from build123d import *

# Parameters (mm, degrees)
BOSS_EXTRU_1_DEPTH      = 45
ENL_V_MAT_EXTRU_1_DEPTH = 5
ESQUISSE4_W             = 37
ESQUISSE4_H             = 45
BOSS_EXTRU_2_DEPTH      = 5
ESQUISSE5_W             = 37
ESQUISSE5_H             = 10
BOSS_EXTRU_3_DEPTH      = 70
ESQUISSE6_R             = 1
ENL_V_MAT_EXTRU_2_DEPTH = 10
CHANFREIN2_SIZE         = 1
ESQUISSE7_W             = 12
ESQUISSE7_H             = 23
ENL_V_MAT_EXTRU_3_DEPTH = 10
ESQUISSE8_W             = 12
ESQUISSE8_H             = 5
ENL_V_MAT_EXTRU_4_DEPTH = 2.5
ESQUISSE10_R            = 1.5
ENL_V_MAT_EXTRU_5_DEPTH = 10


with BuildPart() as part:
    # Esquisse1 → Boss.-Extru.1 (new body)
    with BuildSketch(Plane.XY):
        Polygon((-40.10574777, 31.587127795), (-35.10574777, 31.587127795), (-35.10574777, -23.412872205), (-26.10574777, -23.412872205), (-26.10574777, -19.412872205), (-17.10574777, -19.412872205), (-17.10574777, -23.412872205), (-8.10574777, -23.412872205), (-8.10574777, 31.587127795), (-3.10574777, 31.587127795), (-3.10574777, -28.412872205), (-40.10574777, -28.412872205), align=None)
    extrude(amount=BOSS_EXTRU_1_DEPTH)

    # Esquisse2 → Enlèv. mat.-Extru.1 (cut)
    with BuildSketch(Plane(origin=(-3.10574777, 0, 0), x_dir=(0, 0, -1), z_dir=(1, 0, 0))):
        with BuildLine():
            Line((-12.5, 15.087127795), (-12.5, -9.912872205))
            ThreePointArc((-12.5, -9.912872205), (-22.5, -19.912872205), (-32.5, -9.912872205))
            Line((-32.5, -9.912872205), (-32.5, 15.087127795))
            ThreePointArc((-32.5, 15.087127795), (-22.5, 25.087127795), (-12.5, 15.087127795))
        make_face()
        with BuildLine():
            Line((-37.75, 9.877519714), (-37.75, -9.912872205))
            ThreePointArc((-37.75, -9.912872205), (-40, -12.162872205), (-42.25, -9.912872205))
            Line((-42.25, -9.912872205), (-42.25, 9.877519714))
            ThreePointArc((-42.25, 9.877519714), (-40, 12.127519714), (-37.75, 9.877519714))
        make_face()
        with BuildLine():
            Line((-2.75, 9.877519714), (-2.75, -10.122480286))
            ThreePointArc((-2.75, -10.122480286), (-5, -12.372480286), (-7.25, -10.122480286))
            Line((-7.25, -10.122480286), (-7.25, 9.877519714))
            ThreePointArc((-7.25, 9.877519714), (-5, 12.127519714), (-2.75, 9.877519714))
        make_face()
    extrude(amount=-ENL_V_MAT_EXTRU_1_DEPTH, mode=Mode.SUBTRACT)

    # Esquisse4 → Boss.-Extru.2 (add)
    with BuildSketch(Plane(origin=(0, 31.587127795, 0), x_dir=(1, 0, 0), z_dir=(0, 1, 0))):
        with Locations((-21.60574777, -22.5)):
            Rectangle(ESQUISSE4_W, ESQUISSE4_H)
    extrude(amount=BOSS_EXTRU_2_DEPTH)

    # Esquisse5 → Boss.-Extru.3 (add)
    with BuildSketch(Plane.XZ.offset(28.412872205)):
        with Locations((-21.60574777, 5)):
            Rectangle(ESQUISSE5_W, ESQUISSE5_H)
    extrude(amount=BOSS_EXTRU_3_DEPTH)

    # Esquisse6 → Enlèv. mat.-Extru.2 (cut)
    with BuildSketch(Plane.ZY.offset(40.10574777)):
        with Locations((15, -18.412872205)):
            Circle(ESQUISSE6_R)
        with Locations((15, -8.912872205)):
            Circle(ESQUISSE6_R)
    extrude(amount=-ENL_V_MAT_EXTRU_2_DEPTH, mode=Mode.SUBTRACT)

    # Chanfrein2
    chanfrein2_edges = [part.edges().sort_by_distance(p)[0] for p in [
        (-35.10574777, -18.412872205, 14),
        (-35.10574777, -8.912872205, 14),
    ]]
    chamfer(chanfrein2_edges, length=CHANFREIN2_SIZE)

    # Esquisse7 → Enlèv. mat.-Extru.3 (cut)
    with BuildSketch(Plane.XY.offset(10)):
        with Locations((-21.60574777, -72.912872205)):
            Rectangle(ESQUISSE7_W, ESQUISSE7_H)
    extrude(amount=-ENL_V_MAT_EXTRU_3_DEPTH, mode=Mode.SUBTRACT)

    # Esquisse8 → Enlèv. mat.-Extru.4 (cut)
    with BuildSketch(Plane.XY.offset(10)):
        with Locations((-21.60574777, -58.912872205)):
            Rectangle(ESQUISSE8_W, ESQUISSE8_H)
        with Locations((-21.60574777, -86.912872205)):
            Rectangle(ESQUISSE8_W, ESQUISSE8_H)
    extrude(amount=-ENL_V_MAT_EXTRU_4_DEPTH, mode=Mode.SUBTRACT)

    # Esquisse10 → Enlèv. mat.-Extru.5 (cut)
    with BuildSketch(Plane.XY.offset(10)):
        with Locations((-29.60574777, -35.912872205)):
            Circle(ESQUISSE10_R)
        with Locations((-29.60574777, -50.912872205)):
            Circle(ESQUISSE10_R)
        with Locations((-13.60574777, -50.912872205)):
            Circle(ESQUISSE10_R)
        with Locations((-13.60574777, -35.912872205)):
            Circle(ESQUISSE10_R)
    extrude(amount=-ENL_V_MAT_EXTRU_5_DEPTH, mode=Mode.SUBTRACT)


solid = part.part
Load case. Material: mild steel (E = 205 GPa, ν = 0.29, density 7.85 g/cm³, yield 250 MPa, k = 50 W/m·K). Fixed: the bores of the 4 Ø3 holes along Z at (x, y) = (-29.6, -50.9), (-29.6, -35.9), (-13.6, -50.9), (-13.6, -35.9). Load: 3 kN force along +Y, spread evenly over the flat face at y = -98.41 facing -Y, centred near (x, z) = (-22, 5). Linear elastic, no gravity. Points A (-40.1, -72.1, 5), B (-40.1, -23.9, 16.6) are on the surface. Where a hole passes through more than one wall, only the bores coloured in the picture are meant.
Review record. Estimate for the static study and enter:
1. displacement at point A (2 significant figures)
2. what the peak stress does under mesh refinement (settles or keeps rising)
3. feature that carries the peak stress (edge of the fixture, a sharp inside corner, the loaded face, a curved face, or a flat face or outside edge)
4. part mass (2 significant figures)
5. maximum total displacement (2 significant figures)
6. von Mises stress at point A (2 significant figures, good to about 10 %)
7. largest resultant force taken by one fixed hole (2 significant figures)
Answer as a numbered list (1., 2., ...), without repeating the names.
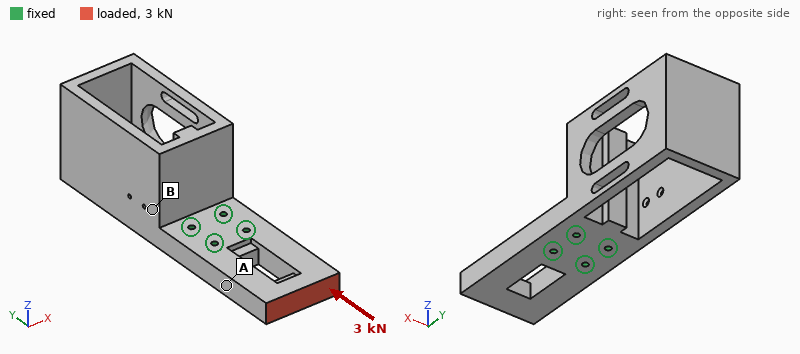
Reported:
1. 1.7 µm
2. keeps rising
3. edge of the fixture
4. 470 g
5. 3.5 µm
6. 7.2 MPa
7. 1.1 kN
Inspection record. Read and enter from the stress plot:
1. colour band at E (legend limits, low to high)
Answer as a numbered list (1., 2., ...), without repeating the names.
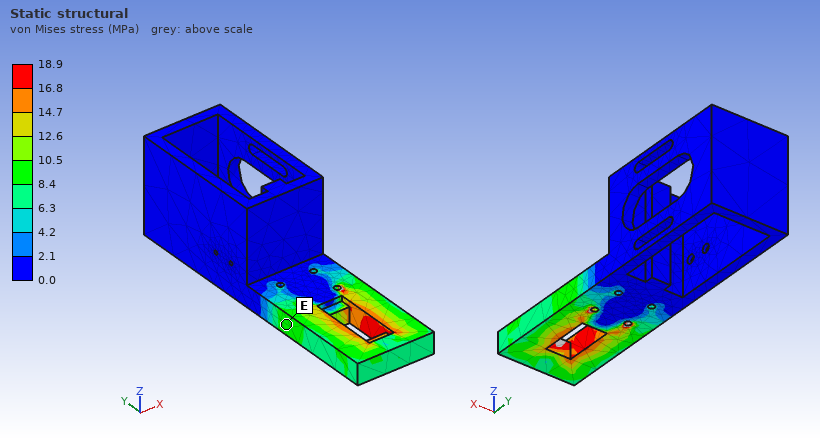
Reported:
1. 8.4 to 10.5 MPa
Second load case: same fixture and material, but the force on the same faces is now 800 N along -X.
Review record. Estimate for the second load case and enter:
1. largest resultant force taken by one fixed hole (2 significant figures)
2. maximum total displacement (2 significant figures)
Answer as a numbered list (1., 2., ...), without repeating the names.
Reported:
1. 1.2 kN
2. 13 µm
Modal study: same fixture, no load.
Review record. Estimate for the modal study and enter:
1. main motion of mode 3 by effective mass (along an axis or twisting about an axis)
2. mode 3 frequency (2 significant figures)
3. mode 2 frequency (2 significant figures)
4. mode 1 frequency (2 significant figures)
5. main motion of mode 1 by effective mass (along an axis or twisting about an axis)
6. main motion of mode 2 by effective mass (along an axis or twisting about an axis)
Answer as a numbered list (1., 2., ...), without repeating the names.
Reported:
1. twisting about Y
2. 2200 Hz
3. 1100 Hz
4. 1000 Hz
5. along Z
6. along X
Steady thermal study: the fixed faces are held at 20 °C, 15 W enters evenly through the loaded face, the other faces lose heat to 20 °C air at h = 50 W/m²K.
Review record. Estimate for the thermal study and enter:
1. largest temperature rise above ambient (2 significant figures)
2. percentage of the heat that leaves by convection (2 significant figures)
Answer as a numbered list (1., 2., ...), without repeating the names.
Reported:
1. 42 K
2. 32 %
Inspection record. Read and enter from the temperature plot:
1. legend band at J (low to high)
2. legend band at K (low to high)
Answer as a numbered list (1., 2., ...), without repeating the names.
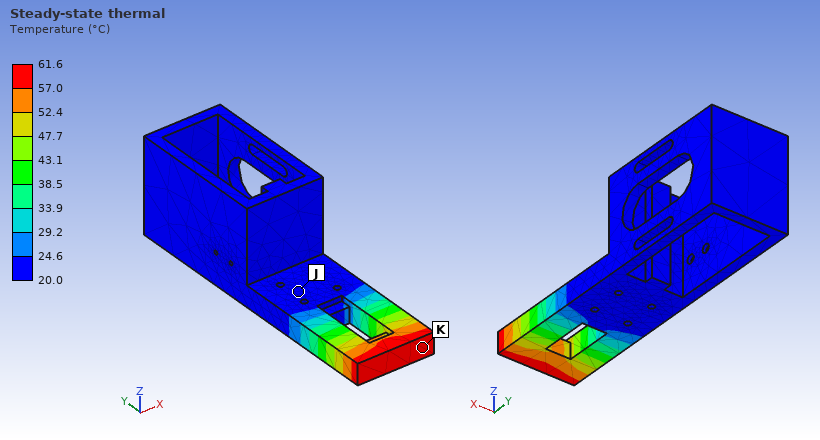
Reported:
1. 20.0 to 24.6 °C
2. 57.0 to 61.6 °C
